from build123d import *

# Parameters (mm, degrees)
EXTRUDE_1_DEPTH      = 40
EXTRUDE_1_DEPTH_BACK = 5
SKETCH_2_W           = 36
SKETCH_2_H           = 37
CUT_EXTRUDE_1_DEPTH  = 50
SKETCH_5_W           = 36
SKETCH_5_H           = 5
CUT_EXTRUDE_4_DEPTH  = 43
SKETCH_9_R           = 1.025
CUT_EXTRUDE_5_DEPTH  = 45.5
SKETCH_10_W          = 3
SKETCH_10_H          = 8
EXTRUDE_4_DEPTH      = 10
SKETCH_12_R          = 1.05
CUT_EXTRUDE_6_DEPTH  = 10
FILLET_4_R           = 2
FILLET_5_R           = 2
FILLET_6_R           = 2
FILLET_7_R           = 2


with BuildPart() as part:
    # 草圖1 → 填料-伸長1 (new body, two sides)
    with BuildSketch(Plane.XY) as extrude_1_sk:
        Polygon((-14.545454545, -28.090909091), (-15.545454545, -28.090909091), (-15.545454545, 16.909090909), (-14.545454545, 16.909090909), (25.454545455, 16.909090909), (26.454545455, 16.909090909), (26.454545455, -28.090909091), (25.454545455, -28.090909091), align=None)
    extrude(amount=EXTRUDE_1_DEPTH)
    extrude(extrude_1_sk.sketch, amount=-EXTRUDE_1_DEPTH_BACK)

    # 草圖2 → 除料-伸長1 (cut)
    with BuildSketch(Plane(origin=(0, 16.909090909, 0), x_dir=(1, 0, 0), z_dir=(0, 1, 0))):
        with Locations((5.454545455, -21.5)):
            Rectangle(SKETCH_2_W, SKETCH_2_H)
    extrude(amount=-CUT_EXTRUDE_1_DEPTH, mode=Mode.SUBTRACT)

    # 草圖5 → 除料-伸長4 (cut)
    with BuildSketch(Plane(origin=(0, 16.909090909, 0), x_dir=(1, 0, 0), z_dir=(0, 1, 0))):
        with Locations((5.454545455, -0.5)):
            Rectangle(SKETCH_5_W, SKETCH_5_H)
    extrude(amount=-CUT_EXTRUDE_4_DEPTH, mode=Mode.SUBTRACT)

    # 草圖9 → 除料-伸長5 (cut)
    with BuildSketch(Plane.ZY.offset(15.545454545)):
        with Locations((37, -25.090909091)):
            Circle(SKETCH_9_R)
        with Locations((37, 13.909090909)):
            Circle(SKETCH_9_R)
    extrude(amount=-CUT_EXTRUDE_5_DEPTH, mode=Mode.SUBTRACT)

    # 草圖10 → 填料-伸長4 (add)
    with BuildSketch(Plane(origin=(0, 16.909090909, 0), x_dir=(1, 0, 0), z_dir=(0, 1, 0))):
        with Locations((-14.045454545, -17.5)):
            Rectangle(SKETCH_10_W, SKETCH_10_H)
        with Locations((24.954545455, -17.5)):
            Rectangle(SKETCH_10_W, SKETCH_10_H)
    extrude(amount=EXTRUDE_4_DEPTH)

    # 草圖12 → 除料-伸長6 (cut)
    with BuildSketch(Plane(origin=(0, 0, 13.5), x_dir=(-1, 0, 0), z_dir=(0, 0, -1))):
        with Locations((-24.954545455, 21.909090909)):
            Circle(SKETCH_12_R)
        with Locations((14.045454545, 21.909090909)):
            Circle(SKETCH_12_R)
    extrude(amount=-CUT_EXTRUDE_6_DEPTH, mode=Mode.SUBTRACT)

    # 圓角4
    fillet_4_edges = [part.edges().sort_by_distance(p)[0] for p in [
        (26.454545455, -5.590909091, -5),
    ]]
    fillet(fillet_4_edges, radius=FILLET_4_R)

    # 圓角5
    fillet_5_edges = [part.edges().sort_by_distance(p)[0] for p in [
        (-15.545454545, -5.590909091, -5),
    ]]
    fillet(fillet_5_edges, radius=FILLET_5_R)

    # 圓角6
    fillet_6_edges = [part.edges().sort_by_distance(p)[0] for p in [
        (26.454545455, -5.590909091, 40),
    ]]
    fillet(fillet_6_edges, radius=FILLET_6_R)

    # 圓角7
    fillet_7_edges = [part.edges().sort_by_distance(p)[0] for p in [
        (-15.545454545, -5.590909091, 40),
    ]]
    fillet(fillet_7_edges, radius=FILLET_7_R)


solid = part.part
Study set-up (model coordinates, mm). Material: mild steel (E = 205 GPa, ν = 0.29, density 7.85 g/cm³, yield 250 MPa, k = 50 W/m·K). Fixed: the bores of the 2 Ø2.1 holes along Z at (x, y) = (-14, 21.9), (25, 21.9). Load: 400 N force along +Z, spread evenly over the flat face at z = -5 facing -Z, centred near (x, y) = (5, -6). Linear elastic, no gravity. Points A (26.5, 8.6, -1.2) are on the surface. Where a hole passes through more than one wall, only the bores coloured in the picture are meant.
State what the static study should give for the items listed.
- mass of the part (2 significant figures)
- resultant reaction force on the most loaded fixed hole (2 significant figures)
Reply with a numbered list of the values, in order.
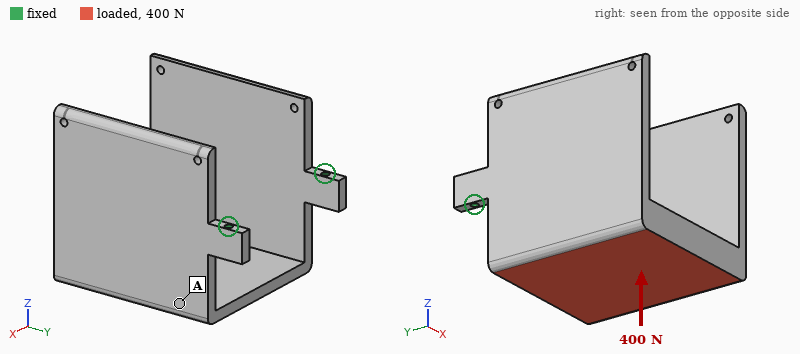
1. 140 g
2. 200 N
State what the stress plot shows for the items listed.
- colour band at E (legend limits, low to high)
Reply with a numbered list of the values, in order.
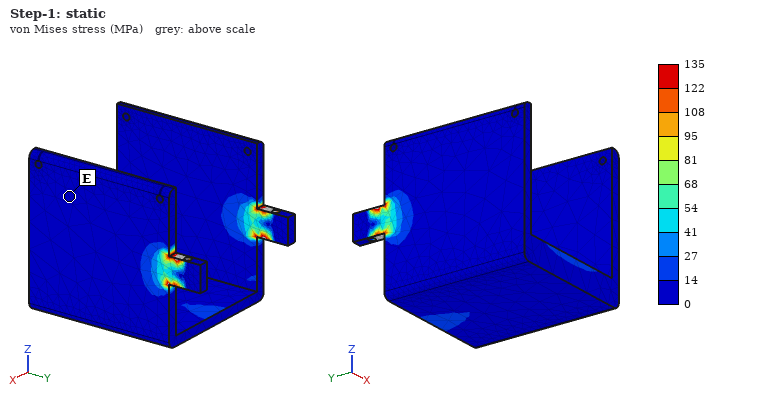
1. 0 to 14 MPa
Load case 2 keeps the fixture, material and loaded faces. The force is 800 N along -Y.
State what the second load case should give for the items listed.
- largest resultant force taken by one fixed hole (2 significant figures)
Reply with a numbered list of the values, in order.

1. 400 N
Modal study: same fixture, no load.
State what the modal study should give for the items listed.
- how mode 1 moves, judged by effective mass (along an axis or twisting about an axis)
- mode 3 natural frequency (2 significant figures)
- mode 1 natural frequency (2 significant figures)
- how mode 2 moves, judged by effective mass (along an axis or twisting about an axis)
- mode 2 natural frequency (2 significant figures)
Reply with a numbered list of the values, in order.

1. along X
2. 1700 Hz
3. 1000 Hz
4. along Z
5. 1200 Hz
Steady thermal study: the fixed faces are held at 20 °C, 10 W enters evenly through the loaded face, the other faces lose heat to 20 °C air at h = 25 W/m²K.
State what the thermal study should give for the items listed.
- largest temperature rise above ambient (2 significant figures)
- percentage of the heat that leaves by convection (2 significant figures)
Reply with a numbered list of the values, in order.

1. 33 K
2. 57 %
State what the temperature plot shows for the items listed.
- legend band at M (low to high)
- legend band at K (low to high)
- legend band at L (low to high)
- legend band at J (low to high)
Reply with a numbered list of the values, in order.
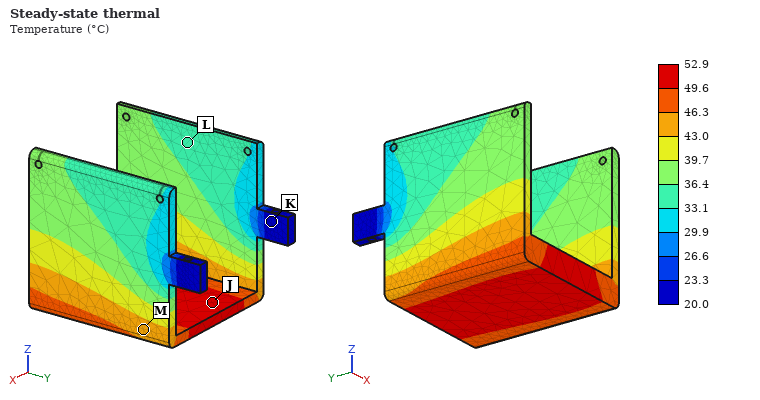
1. 43.0 to 46.3 °C
2. 20.0 to 23.3 °C
3. 33.1 to 36.4 °C
4. 49.6 to 52.9 °C
